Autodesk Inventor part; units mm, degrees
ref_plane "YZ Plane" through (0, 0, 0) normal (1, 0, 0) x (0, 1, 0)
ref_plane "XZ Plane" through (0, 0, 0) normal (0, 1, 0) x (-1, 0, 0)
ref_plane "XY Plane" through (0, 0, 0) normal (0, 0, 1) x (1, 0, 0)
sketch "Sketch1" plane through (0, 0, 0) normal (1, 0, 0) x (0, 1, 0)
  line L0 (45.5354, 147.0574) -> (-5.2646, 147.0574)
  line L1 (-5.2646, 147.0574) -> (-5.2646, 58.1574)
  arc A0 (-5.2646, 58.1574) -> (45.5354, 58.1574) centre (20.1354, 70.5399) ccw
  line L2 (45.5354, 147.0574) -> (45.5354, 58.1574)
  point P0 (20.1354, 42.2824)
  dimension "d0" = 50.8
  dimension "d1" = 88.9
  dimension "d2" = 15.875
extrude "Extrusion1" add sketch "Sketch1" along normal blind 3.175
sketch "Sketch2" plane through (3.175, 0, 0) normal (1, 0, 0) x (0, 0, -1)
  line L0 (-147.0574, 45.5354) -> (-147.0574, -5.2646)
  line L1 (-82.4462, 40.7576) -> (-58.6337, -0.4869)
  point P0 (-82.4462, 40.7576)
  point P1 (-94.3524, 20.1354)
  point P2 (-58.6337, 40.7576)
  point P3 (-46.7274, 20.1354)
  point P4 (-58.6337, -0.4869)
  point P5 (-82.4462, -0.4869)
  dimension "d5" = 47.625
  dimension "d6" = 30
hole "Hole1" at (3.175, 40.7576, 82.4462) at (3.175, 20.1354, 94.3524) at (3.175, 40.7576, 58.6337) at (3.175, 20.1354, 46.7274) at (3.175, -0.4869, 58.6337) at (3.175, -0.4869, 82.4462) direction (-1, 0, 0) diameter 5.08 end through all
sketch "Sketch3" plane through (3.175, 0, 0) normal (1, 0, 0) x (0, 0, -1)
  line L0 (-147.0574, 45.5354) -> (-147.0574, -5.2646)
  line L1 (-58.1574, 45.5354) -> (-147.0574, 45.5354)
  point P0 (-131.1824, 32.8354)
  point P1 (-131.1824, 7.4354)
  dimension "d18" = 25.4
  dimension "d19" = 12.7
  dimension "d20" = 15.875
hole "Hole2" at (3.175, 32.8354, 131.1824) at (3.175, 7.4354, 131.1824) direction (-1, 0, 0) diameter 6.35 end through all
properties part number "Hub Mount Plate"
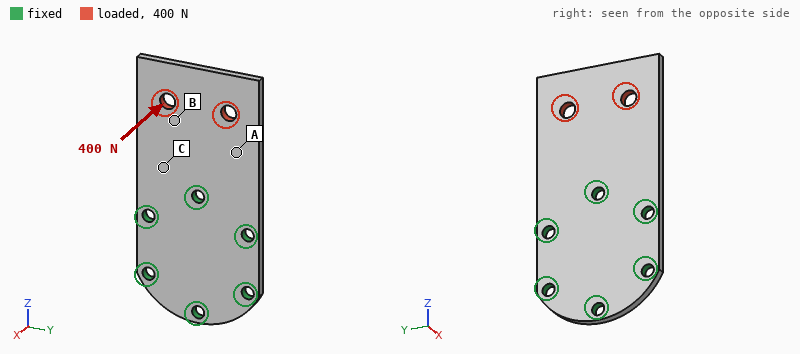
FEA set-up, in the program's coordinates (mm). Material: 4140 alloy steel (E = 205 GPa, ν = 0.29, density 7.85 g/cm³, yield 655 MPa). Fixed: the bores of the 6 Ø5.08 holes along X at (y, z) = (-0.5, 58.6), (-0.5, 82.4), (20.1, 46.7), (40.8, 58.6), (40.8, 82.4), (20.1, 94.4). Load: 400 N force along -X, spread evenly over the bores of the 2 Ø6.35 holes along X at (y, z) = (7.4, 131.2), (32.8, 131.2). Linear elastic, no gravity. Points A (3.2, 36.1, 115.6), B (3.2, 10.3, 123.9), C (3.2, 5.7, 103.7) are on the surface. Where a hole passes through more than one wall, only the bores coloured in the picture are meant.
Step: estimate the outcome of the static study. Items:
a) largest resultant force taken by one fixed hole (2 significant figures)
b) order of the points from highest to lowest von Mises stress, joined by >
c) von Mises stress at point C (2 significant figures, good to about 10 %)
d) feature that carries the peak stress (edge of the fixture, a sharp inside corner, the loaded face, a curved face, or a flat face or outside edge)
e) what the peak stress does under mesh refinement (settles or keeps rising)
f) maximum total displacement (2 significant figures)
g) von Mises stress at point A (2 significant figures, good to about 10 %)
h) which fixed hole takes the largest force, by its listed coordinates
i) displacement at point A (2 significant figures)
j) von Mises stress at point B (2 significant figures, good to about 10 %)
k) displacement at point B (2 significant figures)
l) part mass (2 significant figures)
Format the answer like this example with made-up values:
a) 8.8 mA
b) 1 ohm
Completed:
a) 720 N
b) C > A > B
c) 110 MPa
d) edge of the fixture
e) keeps rising
f) 0.42 mm
g) 71 MPa
h) (20.1, 94.4)
i) 0.12 mm
j) 32 MPa
k) 0.19 mm
l) 120 g
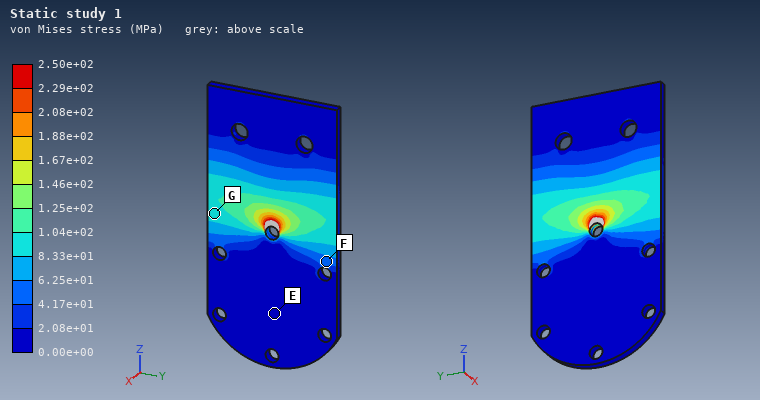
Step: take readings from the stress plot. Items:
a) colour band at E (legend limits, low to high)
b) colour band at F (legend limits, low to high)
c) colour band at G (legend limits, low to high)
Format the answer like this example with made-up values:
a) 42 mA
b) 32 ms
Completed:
a) 0.00e+00 to 2.08e+01 MPa
b) 4.17e+01 to 6.25e+01 MPa
c) 8.33e+01 to 1.04e+02 MPa
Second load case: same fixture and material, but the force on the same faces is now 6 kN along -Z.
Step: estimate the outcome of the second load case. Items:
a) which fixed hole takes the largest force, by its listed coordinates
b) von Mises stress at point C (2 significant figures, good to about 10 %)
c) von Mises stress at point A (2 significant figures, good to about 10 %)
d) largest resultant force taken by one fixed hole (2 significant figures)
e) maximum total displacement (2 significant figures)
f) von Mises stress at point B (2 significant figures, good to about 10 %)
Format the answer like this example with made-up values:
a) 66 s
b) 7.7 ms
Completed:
a) (20.1, 94.4)
b) 32 MPa
c) 38 MPa
d) 2.8 kN
e) 10.0 µm
f) 48 MPa
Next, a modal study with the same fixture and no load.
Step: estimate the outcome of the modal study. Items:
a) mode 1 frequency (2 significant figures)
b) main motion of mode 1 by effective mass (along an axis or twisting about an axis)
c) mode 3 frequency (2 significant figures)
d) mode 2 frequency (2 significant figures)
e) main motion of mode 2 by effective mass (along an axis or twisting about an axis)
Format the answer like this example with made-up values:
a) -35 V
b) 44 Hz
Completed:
a) 920 Hz
b) along X
c) 4900 Hz
d) 2000 Hz
e) twisting about Z
